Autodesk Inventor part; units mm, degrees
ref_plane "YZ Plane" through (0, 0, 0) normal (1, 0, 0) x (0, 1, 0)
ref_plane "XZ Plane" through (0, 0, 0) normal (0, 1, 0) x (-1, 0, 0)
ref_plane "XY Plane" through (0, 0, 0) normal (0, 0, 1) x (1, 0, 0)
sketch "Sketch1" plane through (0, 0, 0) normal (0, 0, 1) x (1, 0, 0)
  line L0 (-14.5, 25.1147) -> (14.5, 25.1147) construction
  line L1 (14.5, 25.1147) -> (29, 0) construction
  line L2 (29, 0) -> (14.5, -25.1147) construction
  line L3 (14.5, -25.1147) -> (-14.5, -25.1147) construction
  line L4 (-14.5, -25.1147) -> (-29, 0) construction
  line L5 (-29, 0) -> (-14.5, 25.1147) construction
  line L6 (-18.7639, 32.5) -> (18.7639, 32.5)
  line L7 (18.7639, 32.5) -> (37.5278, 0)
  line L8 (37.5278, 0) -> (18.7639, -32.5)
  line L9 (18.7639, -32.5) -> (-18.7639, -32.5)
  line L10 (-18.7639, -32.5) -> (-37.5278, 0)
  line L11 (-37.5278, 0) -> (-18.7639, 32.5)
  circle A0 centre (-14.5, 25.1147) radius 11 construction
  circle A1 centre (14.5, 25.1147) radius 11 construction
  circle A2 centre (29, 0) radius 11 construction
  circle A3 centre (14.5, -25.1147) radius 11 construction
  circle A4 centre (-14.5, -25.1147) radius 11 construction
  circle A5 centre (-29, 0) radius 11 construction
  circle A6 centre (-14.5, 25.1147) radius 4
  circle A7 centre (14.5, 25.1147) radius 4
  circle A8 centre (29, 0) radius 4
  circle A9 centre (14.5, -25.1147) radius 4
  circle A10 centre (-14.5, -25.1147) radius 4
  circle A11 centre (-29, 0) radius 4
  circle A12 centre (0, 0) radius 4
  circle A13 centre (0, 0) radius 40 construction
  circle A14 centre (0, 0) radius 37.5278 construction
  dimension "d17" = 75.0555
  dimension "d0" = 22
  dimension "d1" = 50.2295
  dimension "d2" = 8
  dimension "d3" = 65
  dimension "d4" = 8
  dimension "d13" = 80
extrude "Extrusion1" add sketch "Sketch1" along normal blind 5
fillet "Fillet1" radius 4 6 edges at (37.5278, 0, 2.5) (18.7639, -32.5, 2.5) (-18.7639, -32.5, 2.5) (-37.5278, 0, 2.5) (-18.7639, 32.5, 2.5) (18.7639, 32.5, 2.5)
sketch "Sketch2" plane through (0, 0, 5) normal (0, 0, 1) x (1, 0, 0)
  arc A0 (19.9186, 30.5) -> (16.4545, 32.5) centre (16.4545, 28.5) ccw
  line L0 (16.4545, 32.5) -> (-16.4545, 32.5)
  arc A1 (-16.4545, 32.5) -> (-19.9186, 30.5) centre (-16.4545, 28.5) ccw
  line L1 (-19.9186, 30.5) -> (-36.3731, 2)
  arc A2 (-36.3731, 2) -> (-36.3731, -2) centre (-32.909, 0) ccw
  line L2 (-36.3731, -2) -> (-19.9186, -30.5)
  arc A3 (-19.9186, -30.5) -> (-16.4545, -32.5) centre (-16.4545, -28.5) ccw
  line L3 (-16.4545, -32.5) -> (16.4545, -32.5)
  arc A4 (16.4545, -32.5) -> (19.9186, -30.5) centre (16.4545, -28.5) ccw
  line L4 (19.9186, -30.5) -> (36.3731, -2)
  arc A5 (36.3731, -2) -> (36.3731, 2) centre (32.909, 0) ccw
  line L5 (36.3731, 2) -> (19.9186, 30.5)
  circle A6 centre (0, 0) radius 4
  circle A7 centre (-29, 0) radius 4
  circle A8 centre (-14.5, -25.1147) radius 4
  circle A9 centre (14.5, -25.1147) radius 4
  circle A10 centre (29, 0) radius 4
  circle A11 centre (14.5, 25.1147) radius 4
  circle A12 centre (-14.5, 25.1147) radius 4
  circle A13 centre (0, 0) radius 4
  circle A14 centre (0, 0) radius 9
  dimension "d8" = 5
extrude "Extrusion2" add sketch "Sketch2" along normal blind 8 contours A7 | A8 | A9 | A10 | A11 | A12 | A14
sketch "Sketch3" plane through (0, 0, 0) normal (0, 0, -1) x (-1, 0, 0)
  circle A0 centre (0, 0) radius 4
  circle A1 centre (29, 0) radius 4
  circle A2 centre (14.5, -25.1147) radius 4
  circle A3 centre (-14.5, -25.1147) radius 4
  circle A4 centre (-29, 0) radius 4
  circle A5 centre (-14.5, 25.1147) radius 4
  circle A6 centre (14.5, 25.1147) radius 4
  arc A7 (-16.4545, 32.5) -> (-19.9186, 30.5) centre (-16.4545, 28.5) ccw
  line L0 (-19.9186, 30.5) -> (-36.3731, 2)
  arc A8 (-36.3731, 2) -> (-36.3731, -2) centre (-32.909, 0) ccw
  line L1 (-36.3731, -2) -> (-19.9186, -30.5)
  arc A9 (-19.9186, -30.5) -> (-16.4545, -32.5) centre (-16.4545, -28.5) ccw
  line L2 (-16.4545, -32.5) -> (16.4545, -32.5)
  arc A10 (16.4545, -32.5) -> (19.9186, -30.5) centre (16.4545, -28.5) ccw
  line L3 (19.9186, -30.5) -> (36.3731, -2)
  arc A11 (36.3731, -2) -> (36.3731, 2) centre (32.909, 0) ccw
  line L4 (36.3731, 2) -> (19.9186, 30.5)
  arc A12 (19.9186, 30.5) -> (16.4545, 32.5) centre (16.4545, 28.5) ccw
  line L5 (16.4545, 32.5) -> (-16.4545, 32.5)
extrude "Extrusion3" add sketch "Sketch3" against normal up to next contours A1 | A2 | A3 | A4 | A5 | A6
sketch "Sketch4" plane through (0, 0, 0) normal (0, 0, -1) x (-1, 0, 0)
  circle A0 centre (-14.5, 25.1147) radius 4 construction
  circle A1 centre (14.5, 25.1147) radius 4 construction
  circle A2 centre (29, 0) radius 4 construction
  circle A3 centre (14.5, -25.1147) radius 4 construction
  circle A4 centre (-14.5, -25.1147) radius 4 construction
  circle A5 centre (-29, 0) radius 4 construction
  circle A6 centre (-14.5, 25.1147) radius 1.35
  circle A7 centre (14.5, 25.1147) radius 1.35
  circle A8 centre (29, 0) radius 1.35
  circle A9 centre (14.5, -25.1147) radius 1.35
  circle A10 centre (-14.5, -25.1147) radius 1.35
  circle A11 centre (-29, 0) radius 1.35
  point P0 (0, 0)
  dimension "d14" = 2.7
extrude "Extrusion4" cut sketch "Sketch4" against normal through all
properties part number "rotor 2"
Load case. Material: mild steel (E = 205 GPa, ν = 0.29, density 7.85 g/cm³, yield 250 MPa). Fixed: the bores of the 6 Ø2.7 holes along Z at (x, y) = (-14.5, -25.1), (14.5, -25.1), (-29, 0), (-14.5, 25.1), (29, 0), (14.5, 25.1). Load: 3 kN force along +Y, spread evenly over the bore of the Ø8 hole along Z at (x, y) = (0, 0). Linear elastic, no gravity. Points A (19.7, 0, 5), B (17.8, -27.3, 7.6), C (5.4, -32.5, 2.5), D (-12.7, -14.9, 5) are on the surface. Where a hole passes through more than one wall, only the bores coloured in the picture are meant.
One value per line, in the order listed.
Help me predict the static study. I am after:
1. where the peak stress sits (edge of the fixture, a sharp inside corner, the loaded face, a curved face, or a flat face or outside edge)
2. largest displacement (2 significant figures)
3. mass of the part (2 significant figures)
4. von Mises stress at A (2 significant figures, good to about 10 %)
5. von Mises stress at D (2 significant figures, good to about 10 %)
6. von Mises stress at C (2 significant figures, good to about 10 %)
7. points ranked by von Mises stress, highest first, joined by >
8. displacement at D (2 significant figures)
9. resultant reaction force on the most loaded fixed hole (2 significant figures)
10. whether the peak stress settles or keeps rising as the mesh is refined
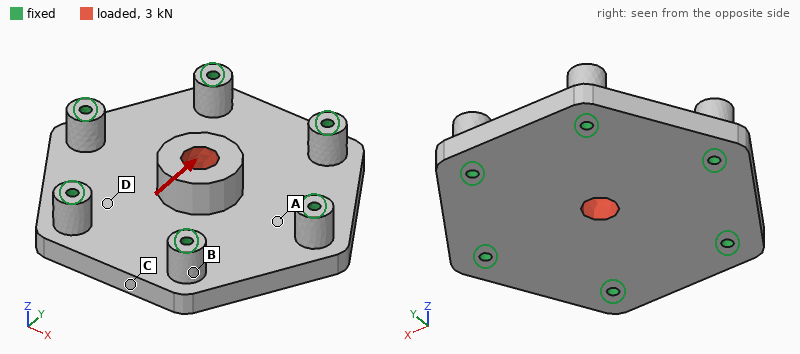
edge of the fixture
5.6 µm
170 g
9.1 MPa
13 MPa
5.0 MPa
D > A > C > B
0.99 µm
680 N
keeps rising
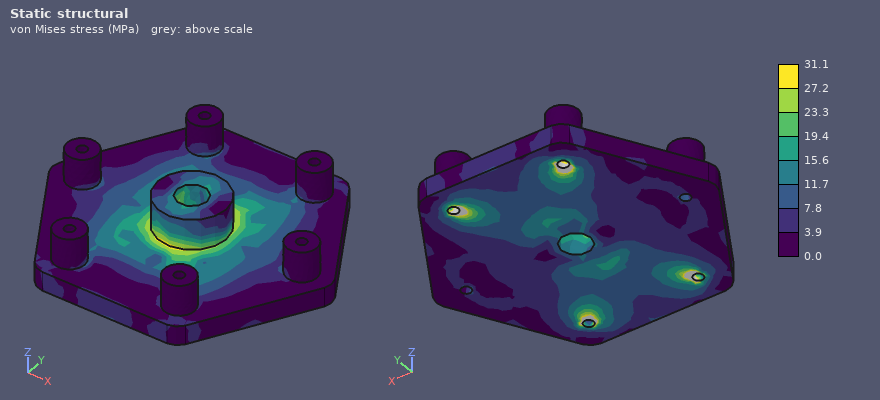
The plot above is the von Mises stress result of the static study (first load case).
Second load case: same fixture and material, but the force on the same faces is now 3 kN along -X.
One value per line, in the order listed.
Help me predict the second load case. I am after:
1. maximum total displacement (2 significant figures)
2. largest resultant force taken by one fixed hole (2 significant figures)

5.6 µm
770 N
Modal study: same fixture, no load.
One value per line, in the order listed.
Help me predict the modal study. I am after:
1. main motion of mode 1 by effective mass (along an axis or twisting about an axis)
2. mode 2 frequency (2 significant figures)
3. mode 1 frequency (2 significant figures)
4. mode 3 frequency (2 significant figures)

along Z
20 kHz
11 kHz
20 kHz
